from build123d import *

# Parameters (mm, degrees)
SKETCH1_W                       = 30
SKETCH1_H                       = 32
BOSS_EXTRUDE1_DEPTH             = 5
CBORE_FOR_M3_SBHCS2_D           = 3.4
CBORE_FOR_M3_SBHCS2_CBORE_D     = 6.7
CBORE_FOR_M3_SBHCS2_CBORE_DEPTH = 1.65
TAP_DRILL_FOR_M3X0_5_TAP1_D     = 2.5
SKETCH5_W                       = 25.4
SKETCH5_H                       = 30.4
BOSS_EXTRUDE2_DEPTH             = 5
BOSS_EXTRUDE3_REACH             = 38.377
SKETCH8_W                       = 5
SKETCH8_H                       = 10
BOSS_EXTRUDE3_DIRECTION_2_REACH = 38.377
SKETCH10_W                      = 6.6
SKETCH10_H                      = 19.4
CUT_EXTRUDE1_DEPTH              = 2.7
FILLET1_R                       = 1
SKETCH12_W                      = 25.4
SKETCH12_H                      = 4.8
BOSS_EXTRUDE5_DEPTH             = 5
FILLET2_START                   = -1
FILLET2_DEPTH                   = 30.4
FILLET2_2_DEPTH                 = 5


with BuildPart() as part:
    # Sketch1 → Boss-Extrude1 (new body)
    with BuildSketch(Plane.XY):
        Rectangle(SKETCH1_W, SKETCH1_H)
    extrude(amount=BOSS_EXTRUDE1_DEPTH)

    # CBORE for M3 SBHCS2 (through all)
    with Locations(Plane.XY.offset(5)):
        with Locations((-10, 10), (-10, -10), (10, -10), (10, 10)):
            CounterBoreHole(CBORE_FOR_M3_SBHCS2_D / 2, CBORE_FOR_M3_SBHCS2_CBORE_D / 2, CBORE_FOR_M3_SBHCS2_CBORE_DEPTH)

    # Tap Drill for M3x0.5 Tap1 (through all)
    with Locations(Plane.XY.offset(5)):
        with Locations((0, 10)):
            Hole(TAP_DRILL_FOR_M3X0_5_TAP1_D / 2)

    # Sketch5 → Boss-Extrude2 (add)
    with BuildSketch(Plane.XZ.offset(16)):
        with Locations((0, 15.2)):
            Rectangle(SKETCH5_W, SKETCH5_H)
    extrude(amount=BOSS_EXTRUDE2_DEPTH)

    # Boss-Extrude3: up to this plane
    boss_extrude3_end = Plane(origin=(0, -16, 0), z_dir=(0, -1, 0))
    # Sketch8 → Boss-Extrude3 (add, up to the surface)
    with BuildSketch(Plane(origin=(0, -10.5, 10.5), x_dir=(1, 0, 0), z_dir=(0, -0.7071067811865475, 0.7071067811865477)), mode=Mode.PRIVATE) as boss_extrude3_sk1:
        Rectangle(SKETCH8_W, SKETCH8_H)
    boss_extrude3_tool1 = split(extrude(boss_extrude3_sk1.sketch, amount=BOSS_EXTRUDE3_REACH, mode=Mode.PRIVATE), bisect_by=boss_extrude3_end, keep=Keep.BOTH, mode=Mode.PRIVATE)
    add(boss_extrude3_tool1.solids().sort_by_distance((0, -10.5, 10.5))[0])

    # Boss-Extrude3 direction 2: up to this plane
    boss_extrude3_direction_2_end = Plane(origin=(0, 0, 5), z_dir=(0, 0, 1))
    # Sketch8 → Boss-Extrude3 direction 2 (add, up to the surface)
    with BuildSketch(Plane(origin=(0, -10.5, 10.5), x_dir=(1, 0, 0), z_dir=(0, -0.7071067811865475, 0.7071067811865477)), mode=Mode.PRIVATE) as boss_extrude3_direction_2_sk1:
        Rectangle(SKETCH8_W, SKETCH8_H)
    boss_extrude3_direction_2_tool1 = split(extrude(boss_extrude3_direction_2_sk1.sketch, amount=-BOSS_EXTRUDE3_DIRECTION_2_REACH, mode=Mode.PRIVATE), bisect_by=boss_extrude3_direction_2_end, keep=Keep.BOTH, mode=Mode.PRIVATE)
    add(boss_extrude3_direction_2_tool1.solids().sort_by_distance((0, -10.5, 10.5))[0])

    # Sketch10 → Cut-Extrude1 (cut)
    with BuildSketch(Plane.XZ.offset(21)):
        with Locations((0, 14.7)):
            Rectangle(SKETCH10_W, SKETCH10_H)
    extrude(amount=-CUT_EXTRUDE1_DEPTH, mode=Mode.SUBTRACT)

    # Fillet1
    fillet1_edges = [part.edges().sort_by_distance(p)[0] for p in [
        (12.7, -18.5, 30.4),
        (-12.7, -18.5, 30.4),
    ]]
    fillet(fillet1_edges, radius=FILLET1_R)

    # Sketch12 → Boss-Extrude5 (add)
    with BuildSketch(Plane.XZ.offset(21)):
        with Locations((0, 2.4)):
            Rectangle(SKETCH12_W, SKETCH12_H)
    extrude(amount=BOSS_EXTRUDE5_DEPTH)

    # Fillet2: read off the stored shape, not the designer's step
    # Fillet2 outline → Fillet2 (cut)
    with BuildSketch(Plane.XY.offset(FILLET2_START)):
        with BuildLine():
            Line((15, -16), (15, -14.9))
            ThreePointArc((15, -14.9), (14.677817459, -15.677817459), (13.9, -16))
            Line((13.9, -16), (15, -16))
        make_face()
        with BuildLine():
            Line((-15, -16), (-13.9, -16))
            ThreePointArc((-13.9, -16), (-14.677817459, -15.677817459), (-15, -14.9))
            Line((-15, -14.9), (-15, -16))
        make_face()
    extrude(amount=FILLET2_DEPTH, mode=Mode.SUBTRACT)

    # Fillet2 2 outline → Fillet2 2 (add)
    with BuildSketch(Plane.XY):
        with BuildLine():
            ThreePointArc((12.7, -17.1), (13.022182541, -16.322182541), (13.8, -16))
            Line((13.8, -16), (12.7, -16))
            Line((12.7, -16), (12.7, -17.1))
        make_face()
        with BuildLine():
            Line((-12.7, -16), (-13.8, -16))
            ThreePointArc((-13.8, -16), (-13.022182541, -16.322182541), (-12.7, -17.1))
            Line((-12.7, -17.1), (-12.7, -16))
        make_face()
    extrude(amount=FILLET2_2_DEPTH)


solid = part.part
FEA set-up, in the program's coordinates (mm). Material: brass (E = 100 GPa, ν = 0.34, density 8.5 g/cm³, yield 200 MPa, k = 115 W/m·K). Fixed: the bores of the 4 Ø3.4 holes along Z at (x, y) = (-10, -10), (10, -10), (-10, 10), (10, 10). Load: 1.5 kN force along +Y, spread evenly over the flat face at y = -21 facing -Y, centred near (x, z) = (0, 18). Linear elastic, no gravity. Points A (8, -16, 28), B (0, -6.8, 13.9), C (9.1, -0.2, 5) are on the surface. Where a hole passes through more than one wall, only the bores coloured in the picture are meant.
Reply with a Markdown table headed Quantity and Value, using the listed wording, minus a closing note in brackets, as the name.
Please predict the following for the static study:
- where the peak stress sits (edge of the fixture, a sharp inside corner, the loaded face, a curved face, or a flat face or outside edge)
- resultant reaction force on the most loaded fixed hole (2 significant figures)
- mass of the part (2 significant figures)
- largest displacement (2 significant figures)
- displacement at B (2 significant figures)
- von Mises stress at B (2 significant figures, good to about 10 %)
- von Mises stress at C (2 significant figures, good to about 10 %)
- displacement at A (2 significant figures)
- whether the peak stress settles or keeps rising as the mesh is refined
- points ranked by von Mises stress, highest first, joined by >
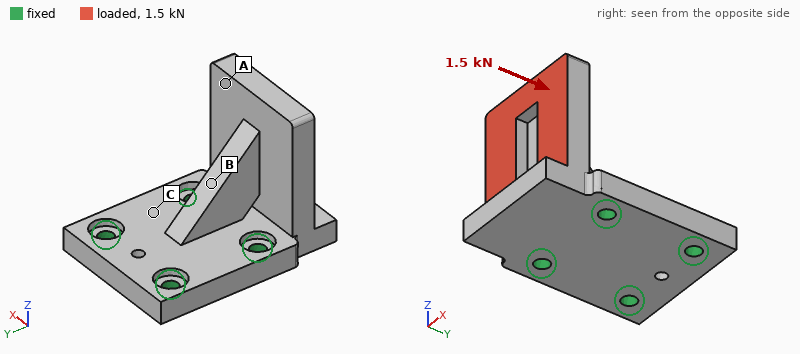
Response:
| Quantity | Value |
|---|---|
| where the peak stress sits | edge of the fixture |
| resultant reaction force on the most loaded fixed hole | 840 N |
| mass of the part | 79 g |
| largest displacement | 93 µm |
| displacement at B | 24 µm |
| von Mises stress at B | 75 MPa |
| von Mises stress at C | 29 MPa |
| displacement at A | 78 µm |
| whether the peak stress settles or keeps rising as the mesh is refined | keeps rising |
| points ranked by von Mises stress, highest first, joined by > | B > C > A |
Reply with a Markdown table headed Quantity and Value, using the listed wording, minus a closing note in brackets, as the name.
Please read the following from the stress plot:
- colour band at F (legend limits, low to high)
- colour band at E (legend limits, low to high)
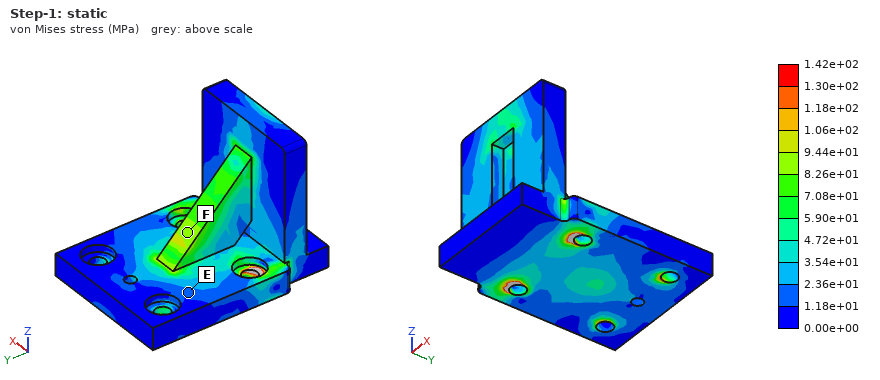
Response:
| Quantity | Value |
|---|---|
| colour band at F | 8.26e+01 to 9.44e+01 MPa |
| colour band at E | 1.18e+01 to 2.36e+01 MPa |
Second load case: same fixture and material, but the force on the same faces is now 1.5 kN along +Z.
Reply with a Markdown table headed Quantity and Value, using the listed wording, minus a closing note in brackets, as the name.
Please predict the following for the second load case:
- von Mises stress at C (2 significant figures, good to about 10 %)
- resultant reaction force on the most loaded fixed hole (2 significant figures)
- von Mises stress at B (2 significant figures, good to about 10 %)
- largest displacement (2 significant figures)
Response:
| Quantity | Value |
|---|---|
| von Mises stress at C | 17 MPa |
| resultant reaction force on the most loaded fixed hole | 1.1 kN |
| von Mises stress at B | 33 MPa |
| largest displacement | 57 µm |
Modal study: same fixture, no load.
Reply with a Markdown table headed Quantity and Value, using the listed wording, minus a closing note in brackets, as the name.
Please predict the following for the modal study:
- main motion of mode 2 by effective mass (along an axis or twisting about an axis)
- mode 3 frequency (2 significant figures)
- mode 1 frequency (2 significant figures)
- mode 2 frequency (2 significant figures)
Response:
| Quantity | Value |
|---|---|
| main motion of mode 2 by effective mass | along X |
| mode 3 frequency | 8000 Hz |
| mode 1 frequency | 4500 Hz |
| mode 2 frequency | 6300 Hz |
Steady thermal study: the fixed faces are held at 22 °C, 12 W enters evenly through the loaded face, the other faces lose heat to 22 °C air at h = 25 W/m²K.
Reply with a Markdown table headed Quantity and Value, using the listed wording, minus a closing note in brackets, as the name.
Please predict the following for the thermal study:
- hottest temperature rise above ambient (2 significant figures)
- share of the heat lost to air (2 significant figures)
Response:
| Quantity | Value |
|---|---|
| hottest temperature rise above ambient | 16 K |
| share of the heat lost to air | 5.1 % |
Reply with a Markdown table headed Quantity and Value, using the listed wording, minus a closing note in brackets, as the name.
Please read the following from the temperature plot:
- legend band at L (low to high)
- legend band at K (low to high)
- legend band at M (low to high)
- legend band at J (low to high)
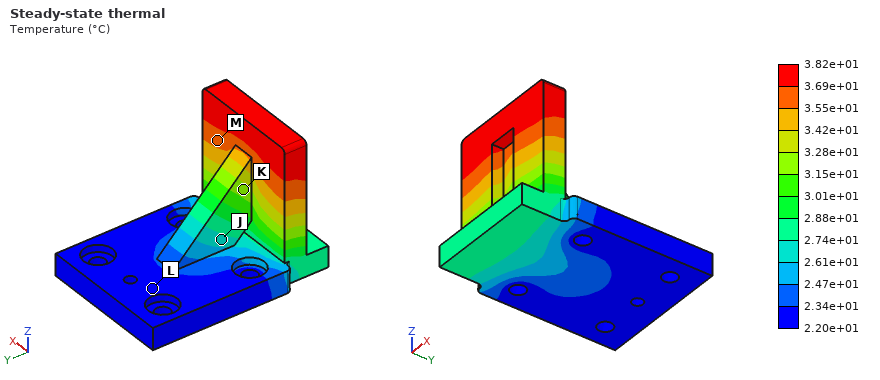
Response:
| Quantity | Value |
|---|---|
| legend band at L | 2.20e+01 to 2.34e+01 °C |
| legend band at K | 3.15e+01 to 3.28e+01 °C |
| legend band at M | 3.55e+01 to 3.69e+01 °C |
| legend band at J | 2.61e+01 to 2.74e+01 °C |
